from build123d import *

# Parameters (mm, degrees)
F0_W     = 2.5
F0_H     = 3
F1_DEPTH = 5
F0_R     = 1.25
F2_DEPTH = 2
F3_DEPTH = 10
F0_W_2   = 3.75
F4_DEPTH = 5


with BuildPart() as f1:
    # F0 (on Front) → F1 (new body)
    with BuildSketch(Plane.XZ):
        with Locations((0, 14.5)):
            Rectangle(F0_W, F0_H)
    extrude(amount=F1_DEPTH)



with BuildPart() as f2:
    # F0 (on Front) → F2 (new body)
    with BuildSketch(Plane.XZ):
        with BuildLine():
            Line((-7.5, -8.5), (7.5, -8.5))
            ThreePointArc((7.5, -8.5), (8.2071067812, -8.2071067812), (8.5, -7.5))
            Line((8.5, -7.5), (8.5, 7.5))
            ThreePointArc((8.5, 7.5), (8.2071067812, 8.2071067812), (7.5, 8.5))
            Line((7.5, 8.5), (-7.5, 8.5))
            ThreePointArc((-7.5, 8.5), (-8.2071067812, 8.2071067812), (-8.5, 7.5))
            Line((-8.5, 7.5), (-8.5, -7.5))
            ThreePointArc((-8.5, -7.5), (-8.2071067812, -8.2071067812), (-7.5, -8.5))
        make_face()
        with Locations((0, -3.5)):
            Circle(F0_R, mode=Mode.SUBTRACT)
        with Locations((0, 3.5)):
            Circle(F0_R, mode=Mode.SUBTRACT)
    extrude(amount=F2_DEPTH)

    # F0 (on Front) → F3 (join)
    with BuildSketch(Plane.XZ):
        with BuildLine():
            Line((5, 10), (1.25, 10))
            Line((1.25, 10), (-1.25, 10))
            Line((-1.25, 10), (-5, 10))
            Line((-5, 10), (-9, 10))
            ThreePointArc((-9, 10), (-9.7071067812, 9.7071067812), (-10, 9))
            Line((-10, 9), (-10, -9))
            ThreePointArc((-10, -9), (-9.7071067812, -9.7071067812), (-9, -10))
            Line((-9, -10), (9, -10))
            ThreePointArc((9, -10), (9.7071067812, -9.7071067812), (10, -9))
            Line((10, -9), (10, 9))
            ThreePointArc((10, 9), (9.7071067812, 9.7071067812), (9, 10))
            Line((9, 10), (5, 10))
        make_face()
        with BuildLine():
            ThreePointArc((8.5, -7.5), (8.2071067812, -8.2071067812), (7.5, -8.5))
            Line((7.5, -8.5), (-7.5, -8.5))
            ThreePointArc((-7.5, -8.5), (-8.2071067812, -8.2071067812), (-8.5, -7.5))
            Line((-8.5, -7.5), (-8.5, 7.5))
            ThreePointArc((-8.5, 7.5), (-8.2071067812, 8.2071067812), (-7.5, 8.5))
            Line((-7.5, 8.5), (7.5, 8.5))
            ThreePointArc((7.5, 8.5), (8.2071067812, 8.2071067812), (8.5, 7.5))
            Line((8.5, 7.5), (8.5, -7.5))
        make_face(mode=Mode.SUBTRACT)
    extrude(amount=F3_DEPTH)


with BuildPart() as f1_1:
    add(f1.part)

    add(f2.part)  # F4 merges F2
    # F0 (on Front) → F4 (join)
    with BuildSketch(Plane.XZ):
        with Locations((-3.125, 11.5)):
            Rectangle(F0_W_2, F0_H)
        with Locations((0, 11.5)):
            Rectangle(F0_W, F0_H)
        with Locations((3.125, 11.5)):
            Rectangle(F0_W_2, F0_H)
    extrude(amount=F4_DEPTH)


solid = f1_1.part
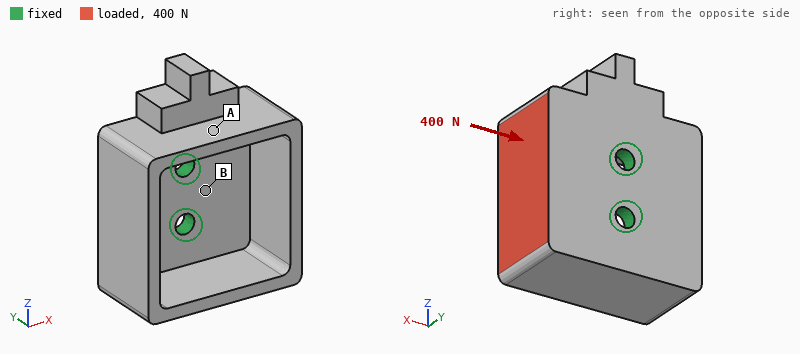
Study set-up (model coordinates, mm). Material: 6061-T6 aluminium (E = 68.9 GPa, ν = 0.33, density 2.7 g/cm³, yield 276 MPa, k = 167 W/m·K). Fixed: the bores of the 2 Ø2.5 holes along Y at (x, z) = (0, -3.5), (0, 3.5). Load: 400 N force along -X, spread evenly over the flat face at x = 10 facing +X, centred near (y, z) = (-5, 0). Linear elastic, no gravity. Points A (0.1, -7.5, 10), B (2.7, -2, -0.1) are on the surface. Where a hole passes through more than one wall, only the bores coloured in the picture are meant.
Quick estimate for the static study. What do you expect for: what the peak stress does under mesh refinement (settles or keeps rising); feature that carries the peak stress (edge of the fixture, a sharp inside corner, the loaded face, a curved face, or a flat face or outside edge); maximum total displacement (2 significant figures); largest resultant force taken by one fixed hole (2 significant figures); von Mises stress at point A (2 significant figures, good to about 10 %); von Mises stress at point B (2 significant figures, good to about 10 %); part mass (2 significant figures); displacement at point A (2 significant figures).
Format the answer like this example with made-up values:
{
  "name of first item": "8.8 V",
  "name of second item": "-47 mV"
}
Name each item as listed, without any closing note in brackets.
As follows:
{
  "what the peak stress does under mesh refinement": "keeps rising",
  "feature that carries the peak stress": "edge of the fixture",
  "maximum total displacement": "68 µm",
  "largest resultant force taken by one fixed hole": "210 N",
  "von Mises stress at point A": "14 MPa",
  "von Mises stress at point B": "46 MPa",
  "part mass": "5.0 g",
  "displacement at point A": "19 µm"
}
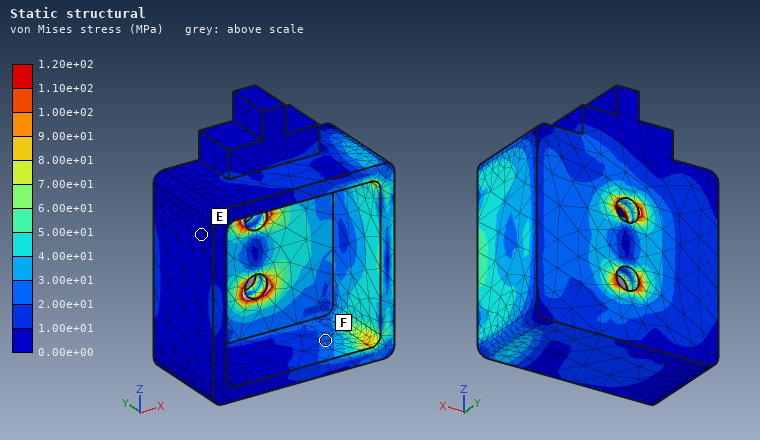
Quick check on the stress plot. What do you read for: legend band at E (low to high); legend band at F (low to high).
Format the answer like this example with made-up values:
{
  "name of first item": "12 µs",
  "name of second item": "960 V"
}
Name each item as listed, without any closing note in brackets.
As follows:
{
  "legend band at E": "0.00e+00 to 1.00e+01 MPa",
  "legend band at F": "2.00e+01 to 3.00e+01 MPa"
}
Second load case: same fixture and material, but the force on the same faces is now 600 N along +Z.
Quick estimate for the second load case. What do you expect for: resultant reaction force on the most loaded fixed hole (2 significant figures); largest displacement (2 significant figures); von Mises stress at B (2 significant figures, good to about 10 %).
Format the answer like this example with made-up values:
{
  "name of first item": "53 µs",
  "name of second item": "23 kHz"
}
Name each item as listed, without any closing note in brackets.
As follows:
{
  "resultant reaction force on the most loaded fixed hole": "740 N",
  "largest displacement": "60 µm",
  "von Mises stress at B": "84 MPa"
}
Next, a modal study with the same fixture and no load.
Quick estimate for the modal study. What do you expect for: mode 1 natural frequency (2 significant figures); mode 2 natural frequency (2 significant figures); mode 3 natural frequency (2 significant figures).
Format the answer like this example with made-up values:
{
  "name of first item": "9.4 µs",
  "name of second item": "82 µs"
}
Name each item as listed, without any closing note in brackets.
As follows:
{
  "mode 1 natural frequency": "7800 Hz",
  "mode 2 natural frequency": "11 kHz",
  "mode 3 natural frequency": "11 kHz"
}
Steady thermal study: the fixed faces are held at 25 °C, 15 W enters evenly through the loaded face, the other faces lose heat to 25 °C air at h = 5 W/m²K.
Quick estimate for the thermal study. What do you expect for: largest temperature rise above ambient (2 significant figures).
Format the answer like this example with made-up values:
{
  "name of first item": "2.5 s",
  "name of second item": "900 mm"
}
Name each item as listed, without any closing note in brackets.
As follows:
{
  "largest temperature rise above ambient": "24 K"
}
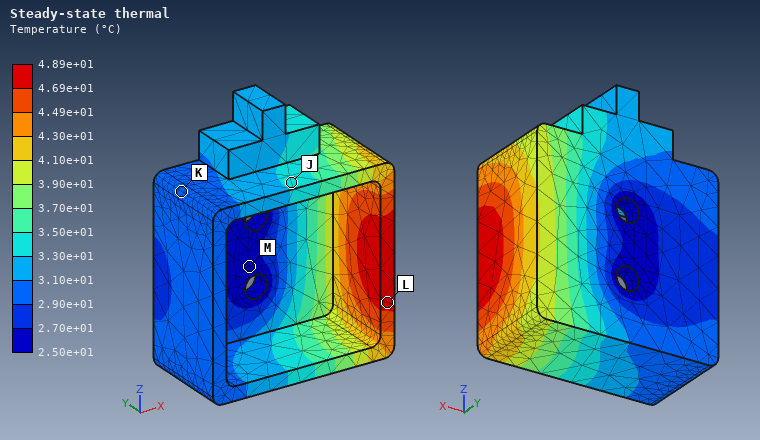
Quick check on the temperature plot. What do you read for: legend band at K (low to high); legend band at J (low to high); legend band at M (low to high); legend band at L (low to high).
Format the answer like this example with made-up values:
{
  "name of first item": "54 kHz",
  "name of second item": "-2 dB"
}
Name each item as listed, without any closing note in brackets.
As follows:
{
  "legend band at K": "2.90e+01 to 3.10e+01 °C",
  "legend band at J": "3.30e+01 to 3.50e+01 °C",
  "legend band at M": "2.50e+01 to 2.70e+01 °C",
  "legend band at L": "4.69e+01 to 4.89e+01 °C"
}
